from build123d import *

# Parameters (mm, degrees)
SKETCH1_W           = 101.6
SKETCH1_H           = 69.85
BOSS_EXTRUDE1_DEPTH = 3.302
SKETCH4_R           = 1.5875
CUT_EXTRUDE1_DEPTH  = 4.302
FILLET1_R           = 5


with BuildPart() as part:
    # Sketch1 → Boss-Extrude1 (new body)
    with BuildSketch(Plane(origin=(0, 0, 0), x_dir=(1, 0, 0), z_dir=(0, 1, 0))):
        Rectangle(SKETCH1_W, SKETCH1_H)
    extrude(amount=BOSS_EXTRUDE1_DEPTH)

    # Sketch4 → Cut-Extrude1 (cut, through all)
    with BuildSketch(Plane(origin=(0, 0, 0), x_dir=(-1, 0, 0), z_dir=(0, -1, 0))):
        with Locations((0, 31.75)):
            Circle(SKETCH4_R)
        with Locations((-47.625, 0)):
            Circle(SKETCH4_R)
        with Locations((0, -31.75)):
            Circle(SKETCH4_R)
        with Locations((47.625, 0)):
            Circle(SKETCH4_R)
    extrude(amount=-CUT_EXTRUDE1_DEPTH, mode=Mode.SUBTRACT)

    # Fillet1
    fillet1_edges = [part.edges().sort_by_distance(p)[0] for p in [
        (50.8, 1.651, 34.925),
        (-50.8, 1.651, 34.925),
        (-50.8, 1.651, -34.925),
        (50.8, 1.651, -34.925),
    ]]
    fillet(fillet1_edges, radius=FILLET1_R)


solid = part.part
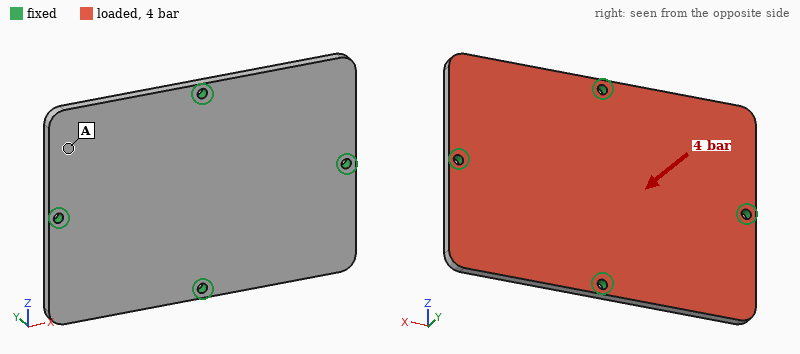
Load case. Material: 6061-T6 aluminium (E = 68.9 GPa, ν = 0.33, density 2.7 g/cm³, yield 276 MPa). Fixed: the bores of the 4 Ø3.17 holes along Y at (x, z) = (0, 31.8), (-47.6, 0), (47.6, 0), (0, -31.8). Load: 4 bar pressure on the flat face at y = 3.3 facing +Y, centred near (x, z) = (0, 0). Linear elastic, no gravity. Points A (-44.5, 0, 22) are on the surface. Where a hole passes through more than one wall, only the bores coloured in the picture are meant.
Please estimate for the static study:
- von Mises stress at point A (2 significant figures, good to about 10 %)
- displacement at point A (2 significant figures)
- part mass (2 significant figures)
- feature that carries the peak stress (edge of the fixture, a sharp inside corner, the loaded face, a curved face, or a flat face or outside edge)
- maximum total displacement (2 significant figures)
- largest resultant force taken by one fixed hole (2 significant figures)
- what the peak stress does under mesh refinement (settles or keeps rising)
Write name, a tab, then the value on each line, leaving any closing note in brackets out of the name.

von Mises stress at point A	25 MPa
displacement at point A	0.100 mm
part mass	63 g
feature that carries the peak stress	edge of the fixture
maximum total displacement	0.17 mm
largest resultant force taken by one fixed hole	720 N
what the peak stress does under mesh refinement	keeps rising
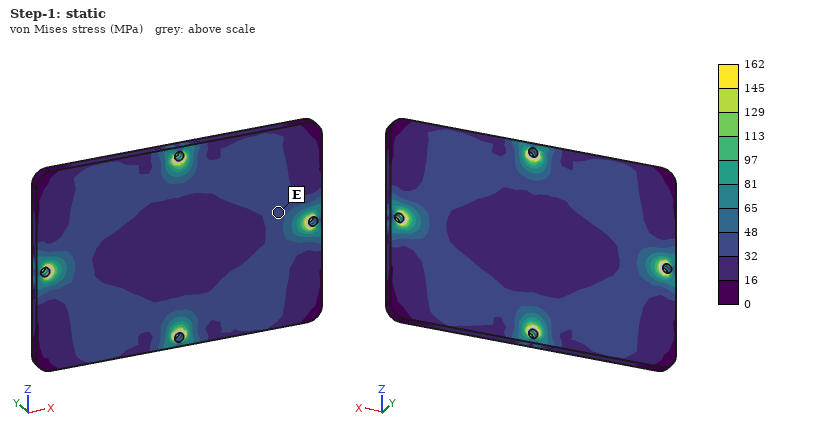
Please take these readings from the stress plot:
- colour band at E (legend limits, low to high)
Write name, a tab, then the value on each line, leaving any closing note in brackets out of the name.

colour band at E	32 to 48 MPa
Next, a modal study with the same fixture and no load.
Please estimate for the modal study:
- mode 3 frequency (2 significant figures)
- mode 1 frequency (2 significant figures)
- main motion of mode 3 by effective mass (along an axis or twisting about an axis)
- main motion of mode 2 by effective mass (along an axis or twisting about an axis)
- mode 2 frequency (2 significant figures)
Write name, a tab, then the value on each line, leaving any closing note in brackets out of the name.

mode 3 frequency	3200 Hz
mode 1 frequency	2800 Hz
main motion of mode 3 by effective mass	twisting about Z
main motion of mode 2 by effective mass	twisting about X
mode 2 frequency	2900 Hz
